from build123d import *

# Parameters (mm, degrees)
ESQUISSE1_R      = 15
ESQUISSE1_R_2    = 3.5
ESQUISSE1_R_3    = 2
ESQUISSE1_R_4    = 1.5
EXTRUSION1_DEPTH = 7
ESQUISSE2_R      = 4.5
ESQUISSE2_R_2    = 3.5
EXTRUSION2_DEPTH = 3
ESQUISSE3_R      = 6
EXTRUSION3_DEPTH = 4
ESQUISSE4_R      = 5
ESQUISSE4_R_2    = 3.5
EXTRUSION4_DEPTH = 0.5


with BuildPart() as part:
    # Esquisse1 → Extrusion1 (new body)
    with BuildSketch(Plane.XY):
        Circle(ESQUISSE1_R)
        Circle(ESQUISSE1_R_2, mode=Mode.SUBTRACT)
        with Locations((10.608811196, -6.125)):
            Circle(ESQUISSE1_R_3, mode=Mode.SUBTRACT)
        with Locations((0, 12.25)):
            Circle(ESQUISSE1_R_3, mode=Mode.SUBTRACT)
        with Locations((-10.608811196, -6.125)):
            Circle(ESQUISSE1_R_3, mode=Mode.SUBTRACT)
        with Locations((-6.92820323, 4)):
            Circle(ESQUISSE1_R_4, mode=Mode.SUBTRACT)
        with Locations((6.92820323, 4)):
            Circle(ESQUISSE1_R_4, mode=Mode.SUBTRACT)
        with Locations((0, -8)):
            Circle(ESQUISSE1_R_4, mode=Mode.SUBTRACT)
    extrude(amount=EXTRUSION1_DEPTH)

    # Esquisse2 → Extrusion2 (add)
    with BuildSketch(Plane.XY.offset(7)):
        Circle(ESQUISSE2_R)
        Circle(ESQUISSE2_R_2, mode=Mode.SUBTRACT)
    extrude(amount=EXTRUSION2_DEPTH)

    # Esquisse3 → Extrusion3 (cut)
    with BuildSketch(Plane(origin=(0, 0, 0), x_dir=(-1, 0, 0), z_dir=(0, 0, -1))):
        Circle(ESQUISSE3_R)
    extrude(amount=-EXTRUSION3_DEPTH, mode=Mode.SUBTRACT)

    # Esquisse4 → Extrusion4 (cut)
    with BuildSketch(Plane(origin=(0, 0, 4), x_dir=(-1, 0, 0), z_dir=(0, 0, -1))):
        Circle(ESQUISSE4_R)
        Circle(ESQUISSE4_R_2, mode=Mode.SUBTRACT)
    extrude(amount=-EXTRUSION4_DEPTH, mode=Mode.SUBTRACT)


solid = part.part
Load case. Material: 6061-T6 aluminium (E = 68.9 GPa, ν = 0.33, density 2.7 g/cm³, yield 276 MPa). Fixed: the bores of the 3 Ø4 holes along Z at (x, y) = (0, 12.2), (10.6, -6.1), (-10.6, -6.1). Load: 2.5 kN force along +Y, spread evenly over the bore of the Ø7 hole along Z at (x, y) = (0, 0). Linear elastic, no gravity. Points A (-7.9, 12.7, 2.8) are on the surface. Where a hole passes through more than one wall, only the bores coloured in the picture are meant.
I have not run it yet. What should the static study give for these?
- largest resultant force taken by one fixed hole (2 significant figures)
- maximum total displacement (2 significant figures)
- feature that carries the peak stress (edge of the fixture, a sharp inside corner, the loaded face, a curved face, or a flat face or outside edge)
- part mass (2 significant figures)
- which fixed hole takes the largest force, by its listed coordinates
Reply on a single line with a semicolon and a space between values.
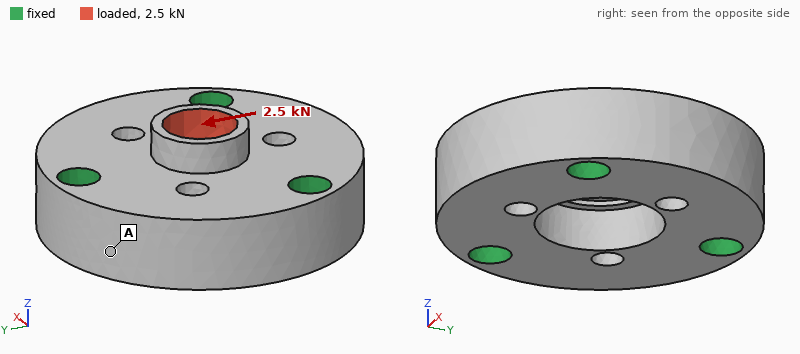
950 N; 20 µm; the loaded face; 11 g; (0, 12.2)
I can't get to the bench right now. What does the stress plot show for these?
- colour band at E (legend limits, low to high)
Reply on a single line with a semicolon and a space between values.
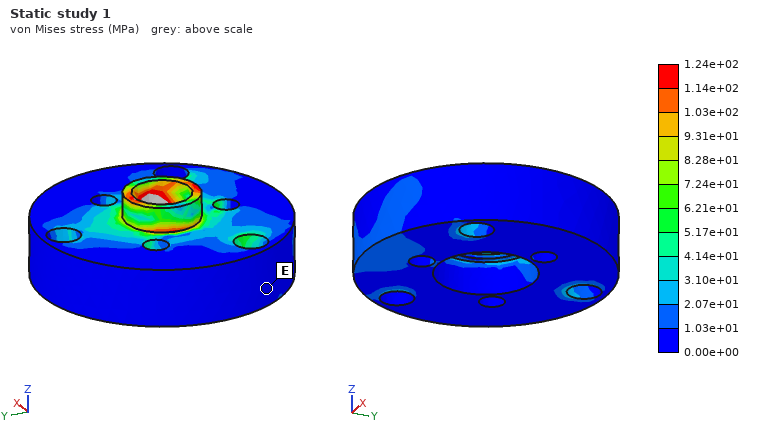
0.00e+00 to 1.03e+01 MPa
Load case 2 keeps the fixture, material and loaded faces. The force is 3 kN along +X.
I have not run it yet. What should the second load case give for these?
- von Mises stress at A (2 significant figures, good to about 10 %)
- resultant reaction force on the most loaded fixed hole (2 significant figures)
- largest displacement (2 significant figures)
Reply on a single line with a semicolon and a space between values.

11 MPa; 1.1 kN; 22 µm
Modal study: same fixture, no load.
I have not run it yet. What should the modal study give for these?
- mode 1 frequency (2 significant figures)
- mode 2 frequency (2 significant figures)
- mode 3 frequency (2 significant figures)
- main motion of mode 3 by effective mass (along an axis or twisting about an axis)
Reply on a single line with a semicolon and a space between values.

44 kHz; 44 kHz; 48 kHz; along Z
